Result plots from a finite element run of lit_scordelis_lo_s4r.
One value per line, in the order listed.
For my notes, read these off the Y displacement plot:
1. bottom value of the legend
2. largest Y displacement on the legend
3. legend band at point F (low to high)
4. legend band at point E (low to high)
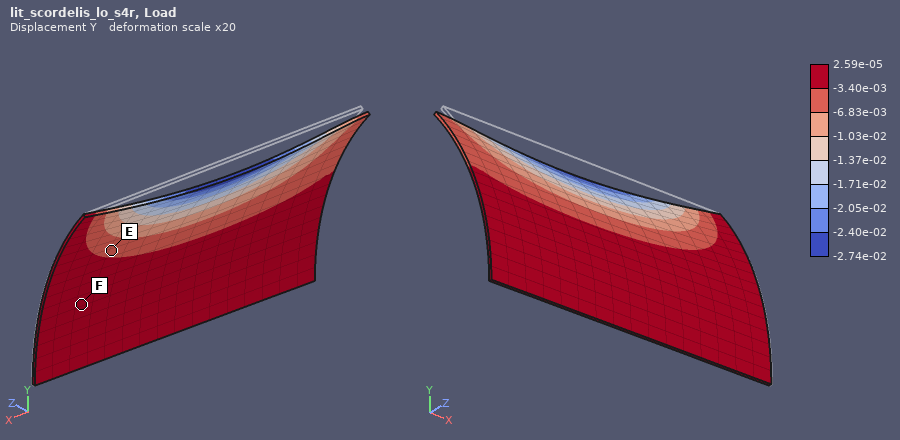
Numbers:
-2.74e-02
2.59e-05
-3.40e-03 to 2.59e-05
-6.83e-03 to -3.40e-03
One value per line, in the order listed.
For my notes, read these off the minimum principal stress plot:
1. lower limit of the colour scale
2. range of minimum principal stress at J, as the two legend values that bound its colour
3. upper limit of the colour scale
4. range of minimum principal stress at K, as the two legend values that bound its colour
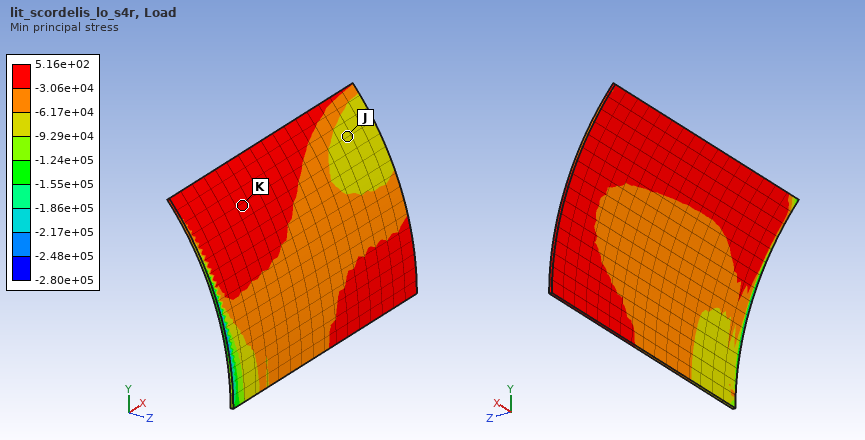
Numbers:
-2.80e+05
-9.29e+04 to -6.17e+04
5.16e+02
-3.06e+04 to 5.16e+02
